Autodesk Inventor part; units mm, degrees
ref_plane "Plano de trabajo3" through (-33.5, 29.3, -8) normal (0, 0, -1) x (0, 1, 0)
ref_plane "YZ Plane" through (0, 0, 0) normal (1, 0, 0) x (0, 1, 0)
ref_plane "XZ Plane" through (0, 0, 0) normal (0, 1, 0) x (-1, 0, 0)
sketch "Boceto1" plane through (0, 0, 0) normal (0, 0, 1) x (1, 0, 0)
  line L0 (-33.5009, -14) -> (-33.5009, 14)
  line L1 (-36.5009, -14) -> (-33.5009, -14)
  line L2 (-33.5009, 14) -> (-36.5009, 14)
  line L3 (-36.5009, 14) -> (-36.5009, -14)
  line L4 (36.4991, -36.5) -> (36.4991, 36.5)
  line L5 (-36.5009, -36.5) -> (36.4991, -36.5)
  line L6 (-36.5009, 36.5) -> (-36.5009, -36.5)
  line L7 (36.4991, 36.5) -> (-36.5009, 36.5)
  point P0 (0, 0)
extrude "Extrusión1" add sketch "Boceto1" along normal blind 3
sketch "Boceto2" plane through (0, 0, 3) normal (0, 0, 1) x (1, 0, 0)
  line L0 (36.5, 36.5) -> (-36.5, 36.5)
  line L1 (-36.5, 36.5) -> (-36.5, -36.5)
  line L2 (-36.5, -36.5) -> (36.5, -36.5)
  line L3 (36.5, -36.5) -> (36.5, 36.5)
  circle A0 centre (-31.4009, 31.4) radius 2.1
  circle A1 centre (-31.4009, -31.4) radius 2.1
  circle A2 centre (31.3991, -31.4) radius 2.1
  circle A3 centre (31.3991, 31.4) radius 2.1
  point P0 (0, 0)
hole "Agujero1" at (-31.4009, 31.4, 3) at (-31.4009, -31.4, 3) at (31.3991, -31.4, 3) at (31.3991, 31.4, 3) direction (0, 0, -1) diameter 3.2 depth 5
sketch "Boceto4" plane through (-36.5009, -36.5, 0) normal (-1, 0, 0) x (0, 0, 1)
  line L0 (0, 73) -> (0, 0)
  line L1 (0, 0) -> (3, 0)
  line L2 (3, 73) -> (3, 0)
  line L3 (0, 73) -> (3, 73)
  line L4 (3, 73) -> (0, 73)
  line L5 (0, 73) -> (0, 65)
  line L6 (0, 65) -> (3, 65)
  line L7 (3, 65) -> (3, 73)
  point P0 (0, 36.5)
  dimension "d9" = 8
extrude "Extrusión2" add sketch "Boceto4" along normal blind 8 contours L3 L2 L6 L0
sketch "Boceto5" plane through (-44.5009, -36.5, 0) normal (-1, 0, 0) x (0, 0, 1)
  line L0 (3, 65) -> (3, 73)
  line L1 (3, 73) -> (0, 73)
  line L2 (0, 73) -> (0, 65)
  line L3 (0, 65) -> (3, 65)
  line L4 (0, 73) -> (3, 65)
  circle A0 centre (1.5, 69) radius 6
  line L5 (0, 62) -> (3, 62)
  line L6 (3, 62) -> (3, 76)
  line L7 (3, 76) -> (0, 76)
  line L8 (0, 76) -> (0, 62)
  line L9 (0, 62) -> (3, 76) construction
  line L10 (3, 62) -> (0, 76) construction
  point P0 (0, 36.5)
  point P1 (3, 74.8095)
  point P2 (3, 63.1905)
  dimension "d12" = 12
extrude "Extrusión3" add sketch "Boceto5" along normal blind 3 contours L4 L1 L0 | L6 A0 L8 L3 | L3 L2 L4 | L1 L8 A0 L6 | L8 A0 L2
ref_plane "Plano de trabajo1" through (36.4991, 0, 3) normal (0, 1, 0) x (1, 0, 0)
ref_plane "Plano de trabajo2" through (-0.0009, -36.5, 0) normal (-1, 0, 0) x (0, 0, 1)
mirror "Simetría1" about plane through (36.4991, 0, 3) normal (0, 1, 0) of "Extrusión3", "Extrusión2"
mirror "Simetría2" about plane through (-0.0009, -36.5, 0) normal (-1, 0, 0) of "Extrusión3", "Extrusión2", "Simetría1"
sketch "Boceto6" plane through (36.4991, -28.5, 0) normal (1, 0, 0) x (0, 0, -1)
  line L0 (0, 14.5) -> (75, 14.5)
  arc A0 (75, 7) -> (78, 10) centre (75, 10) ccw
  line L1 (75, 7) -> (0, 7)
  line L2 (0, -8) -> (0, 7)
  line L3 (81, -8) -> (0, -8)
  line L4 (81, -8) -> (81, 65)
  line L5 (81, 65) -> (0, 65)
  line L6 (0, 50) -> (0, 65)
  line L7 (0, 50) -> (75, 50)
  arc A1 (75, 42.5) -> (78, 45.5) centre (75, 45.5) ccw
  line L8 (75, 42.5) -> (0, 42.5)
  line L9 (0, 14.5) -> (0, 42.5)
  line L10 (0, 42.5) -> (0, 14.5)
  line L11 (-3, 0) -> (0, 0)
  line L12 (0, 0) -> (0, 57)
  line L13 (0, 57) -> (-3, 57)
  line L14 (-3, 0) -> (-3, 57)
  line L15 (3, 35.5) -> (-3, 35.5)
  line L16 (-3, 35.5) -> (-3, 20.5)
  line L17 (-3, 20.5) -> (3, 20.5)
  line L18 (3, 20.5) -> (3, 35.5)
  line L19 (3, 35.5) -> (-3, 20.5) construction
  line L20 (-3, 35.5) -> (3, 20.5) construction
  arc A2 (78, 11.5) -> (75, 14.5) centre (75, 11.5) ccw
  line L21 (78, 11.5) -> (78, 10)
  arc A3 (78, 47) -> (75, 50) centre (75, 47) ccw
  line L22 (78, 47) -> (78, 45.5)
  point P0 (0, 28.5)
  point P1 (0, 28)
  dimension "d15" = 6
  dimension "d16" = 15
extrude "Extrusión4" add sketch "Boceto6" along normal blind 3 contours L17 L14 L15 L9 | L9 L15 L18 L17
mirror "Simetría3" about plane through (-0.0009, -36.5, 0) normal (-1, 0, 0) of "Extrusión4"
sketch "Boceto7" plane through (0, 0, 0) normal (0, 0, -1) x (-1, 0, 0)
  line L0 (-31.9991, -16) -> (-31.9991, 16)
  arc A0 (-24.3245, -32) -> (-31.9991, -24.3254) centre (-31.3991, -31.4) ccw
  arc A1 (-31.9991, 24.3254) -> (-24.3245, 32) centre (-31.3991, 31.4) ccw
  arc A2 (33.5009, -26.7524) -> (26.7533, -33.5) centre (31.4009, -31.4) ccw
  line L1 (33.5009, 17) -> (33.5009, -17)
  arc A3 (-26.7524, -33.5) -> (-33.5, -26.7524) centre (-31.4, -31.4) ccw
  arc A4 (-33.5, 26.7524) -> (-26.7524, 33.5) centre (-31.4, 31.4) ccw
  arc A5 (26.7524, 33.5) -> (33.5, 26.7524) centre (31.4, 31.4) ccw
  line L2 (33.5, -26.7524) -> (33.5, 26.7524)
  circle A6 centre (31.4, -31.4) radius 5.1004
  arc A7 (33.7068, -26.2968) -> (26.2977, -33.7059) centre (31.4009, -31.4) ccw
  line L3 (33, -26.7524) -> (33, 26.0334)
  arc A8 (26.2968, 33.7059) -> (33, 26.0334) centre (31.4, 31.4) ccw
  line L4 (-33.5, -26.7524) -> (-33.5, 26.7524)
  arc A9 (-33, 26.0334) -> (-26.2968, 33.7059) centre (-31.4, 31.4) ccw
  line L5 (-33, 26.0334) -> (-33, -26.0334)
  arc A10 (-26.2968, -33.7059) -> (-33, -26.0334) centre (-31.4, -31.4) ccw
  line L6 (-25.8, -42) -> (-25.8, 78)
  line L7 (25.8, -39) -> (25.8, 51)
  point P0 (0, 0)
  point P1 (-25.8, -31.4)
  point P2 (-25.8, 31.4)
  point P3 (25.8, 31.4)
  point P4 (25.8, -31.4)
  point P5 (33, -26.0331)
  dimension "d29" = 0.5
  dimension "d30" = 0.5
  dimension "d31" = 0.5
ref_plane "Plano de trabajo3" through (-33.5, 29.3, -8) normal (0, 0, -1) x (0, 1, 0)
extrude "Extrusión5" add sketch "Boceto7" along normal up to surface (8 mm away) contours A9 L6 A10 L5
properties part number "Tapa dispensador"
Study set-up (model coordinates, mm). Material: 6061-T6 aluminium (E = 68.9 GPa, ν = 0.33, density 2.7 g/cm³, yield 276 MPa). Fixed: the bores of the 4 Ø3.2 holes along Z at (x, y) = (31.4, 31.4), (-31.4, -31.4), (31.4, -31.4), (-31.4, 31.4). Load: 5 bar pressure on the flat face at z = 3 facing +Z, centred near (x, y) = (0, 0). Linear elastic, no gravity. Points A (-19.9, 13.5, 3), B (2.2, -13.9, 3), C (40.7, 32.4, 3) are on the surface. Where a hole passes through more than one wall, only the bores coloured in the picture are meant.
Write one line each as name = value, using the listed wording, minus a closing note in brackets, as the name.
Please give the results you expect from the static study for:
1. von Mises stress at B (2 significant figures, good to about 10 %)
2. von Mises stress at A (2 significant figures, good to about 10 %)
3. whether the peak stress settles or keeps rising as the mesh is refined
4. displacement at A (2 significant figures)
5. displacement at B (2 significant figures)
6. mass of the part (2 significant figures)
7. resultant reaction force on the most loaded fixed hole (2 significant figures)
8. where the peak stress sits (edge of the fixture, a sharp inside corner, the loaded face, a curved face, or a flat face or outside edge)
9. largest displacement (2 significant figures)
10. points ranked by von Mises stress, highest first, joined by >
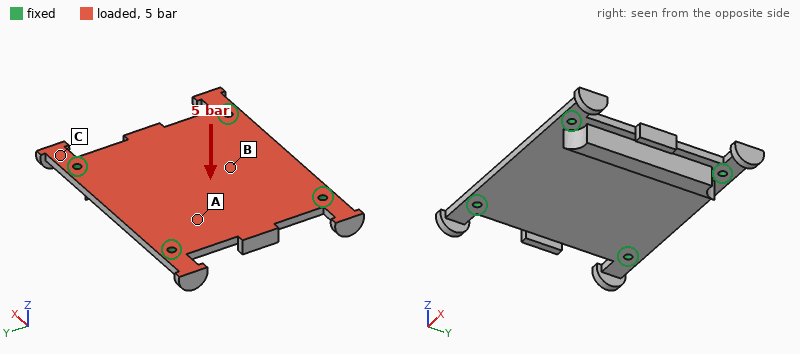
von Mises stress at B = 62 MPa
von Mises stress at A = 43 MPa
whether the peak stress settles or keeps rising as the mesh is refined = keeps rising
displacement at A = 0.19 mm
displacement at B = 0.24 mm
mass of the part = 57 g
resultant reaction force on the most loaded fixed hole = 890 N
where the peak stress sits = edge of the fixture
largest displacement = 0.28 mm
points ranked by von Mises stress, highest first, joined by > = B > A > C
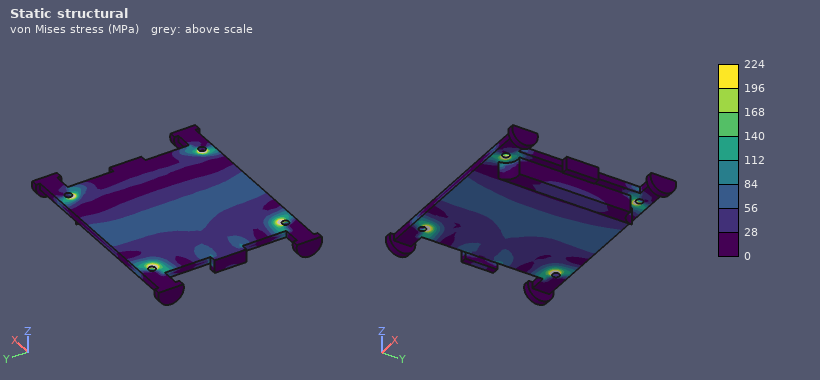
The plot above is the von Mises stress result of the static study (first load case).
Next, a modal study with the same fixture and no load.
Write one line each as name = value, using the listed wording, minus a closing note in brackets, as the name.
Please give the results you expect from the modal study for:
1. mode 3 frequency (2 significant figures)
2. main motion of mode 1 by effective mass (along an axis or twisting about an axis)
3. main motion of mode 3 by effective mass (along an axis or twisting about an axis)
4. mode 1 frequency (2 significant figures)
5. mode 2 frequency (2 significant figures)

mode 3 frequency = 4600 Hz
main motion of mode 1 by effective mass = along Z
main motion of mode 3 by effective mass = twisting about X
mode 1 frequency = 2800 Hz
mode 2 frequency = 4200 Hz
